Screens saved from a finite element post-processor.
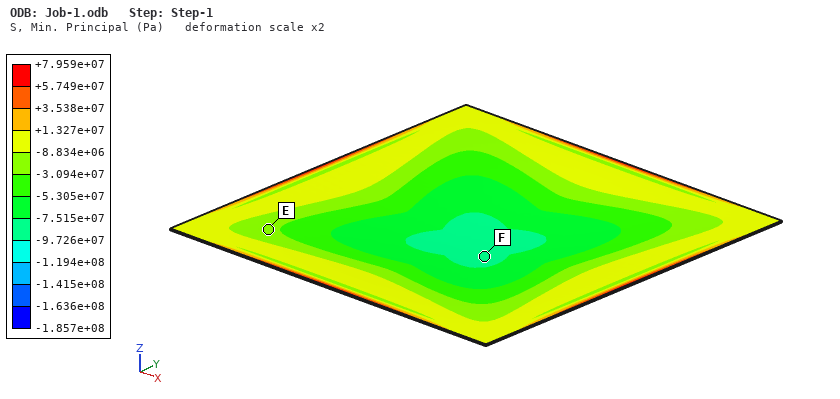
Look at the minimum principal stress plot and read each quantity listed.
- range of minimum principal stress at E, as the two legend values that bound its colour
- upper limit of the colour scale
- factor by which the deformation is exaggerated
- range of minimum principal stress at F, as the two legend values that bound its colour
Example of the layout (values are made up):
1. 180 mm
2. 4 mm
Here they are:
1. -3.094e+07 to -8.834e+06 Pa
2. +7.959e+07 Pa
3. 2
4. -9.726e+07 to -7.515e+07 Pa
